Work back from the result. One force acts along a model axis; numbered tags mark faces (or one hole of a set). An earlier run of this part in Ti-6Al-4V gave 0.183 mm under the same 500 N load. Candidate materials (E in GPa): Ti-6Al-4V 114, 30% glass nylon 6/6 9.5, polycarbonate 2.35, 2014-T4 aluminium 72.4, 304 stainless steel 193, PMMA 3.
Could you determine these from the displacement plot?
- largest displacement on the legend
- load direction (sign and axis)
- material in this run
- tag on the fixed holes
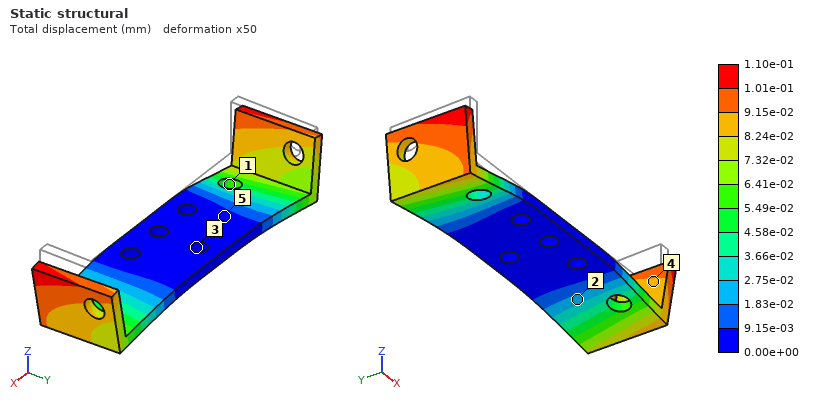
1.10e-01 mm
-Z
304 stainless steel
3
